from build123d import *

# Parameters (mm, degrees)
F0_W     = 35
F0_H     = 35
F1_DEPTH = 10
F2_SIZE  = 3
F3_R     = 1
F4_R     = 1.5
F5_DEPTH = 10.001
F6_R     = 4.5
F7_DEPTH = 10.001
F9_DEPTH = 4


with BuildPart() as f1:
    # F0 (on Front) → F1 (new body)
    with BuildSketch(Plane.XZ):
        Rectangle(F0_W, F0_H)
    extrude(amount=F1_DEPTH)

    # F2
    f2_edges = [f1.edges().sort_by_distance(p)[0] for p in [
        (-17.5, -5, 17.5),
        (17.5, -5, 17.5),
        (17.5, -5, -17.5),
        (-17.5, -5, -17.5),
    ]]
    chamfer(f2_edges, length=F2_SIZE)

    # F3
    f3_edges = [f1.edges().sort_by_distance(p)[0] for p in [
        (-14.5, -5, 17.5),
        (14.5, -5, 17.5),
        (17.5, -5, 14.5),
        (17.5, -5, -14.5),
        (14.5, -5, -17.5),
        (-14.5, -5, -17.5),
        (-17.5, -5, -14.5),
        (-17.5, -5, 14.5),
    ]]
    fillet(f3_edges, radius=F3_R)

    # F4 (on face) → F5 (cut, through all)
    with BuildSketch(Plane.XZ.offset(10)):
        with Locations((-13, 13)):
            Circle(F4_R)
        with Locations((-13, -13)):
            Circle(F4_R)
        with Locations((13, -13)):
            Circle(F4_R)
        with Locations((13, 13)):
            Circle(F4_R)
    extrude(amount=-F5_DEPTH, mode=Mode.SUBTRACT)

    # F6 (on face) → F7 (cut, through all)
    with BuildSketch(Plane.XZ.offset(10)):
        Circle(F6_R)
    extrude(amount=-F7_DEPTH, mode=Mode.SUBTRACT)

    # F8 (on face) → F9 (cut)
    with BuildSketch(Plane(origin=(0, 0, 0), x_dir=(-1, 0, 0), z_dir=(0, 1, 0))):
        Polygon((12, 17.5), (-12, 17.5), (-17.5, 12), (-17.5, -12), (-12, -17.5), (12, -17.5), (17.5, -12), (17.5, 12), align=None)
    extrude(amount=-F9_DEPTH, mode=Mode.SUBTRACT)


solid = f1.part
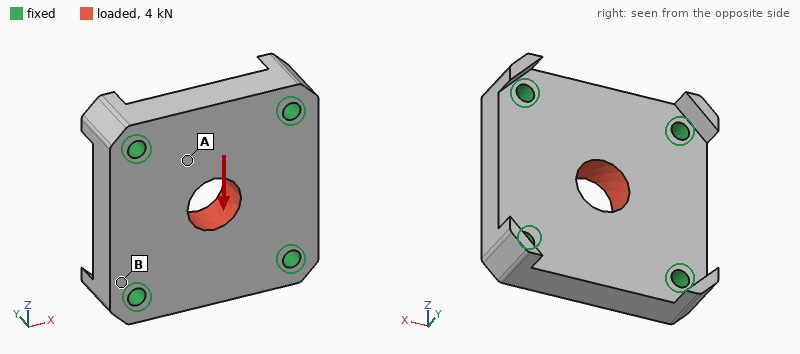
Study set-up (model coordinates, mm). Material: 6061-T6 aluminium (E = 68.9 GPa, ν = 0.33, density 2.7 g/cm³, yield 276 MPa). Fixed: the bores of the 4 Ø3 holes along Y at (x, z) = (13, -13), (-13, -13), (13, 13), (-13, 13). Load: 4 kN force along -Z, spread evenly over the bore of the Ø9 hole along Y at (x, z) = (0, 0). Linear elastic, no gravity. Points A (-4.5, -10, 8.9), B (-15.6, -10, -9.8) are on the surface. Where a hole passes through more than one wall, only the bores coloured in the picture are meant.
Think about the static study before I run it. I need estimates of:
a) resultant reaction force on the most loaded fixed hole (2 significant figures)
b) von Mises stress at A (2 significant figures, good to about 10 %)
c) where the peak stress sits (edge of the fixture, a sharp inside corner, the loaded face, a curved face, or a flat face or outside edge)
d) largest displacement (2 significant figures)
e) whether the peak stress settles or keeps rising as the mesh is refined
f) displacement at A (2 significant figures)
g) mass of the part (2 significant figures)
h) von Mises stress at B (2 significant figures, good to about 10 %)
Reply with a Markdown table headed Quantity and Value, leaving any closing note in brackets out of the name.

| Quantity | Value |
|---|---|
| resultant reaction force on the most loaded fixed hole | 1.1 kN |
| von Mises stress at A | 18 MPa |
| where the peak stress sits | edge of the fixture |
| largest displacement | 6.1 µm |
| whether the peak stress settles or keeps rising as the mesh is refined | keeps rising |
| displacement at A | 4.0 µm |
| mass of the part | 19 g |
| von Mises stress at B | 6.5 MPa |
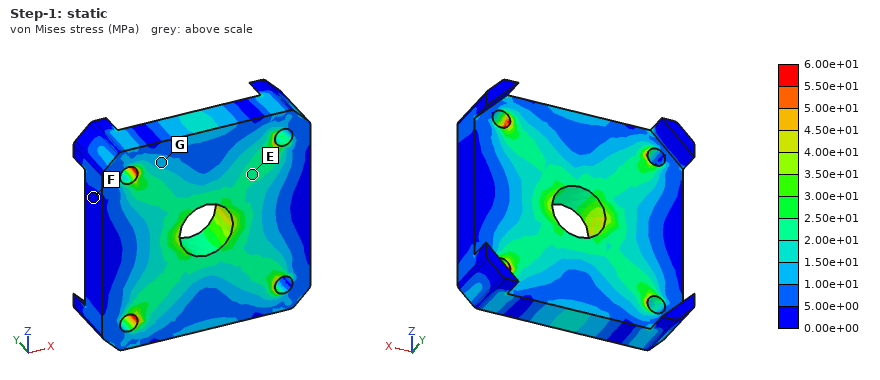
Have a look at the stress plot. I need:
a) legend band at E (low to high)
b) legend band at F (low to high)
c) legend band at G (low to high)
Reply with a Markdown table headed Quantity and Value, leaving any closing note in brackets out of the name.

| Quantity | Value |
|---|---|
| legend band at E | 2.00e+01 to 2.50e+01 MPa |
| legend band at F | 0.00e+00 to 5.00e+00 MPa |
| legend band at G | 1.00e+01 to 1.50e+01 MPa |
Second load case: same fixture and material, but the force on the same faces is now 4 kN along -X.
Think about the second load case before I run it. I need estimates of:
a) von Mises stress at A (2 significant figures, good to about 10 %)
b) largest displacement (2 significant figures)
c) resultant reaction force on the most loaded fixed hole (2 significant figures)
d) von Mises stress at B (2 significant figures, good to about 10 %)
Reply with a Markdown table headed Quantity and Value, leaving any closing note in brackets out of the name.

| Quantity | Value |
|---|---|
| von Mises stress at A | 18 MPa |
| largest displacement | 6.1 µm |
| resultant reaction force on the most loaded fixed hole | 1.1 kN |
| von Mises stress at B | 12 MPa |
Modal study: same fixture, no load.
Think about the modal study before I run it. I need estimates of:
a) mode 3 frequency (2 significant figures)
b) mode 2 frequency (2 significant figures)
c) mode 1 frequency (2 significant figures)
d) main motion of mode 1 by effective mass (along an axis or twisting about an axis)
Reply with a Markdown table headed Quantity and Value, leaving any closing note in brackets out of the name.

| Quantity | Value |
|---|---|
| mode 3 frequency | 38 kHz |
| mode 2 frequency | 38 kHz |
| mode 1 frequency | 27 kHz |
| main motion of mode 1 by effective mass | along Y |
